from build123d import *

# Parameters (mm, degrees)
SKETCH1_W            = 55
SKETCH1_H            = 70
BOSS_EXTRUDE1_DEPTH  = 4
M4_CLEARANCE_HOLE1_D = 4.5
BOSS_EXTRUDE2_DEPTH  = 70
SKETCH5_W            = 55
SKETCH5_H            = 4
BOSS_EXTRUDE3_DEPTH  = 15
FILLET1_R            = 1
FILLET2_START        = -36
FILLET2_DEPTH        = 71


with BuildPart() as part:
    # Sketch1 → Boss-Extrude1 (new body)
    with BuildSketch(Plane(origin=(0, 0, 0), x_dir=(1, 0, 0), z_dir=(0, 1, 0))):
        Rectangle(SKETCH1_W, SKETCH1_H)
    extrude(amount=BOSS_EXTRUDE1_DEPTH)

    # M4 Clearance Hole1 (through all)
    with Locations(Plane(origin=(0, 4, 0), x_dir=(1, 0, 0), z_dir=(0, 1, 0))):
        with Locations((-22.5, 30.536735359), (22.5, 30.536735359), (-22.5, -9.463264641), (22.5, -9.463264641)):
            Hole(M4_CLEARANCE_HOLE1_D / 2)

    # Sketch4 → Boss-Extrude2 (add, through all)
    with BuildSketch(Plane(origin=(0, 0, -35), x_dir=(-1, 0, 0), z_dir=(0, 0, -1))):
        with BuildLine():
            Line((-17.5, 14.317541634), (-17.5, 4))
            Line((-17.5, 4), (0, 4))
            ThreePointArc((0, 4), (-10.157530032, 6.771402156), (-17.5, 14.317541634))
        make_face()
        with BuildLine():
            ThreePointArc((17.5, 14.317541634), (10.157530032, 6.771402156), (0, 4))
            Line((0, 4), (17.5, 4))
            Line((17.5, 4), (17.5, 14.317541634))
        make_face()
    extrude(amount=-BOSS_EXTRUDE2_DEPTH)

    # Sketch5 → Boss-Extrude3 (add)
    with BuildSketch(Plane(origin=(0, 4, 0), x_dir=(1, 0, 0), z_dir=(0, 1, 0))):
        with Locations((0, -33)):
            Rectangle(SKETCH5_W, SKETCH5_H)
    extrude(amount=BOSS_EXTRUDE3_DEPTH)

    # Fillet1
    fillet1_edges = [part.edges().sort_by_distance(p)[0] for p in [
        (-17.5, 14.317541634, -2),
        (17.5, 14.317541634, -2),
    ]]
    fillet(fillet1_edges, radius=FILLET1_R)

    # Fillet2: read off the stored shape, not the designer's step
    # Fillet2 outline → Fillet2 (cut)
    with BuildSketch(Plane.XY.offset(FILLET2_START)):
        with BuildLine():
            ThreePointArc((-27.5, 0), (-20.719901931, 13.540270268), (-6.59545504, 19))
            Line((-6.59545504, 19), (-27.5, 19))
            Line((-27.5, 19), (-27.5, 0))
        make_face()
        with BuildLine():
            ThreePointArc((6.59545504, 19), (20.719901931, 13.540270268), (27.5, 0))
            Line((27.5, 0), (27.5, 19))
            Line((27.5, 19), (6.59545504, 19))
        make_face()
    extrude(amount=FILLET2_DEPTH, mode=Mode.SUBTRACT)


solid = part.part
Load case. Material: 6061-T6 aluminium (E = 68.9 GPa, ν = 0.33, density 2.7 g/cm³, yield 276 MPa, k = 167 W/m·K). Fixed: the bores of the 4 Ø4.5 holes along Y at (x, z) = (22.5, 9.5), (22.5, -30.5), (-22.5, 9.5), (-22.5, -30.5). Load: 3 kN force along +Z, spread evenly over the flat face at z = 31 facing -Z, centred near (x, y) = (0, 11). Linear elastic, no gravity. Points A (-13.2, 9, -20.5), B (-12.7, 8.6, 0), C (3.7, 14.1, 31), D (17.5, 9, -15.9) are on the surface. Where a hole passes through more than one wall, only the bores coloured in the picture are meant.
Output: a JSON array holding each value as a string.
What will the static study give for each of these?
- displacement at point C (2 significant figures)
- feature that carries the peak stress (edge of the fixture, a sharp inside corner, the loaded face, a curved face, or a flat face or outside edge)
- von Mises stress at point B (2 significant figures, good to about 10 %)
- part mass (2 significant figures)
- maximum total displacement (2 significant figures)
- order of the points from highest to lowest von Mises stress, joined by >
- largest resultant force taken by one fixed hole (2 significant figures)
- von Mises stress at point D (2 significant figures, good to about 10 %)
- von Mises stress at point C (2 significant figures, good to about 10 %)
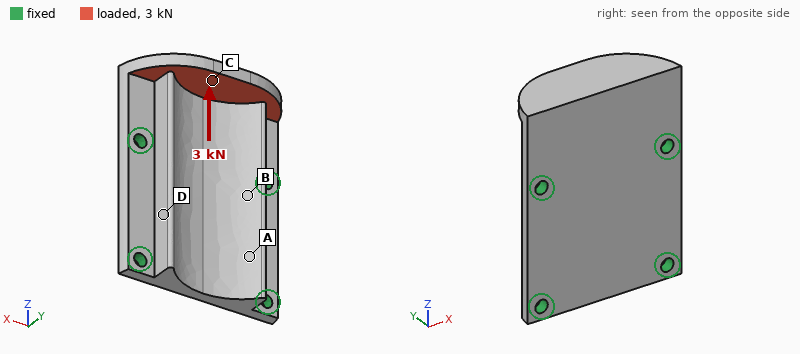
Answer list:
["0.12 mm", "a curved face", "33 MPa", "65 g", "0.19 mm", "C > B > D > A", "830 N", "18 MPa", "47 MPa"]
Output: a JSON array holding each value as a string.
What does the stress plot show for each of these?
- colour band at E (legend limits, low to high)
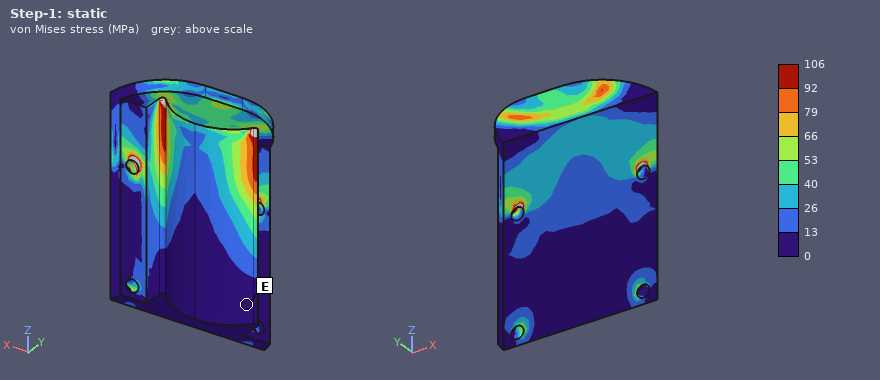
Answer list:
["0 to 13 MPa"]
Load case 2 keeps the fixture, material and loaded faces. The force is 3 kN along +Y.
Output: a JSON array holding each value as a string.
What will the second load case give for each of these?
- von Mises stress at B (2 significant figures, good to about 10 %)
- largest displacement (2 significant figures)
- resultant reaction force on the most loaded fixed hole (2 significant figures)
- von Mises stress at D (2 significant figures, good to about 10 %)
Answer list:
["70 MPa", "0.26 mm", "2.5 kN", "41 MPa"]
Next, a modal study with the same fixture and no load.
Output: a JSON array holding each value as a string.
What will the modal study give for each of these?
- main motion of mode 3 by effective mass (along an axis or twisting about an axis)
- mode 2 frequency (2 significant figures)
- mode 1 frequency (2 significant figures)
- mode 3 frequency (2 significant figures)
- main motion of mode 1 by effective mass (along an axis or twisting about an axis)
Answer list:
["along Y", "7700 Hz", "4600 Hz", "8500 Hz", "along Y"]
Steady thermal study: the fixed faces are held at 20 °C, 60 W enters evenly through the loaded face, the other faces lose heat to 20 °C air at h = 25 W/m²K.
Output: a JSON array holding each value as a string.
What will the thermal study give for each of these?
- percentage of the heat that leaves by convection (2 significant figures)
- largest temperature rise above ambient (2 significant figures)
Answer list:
["5.7 %", "49 K"]
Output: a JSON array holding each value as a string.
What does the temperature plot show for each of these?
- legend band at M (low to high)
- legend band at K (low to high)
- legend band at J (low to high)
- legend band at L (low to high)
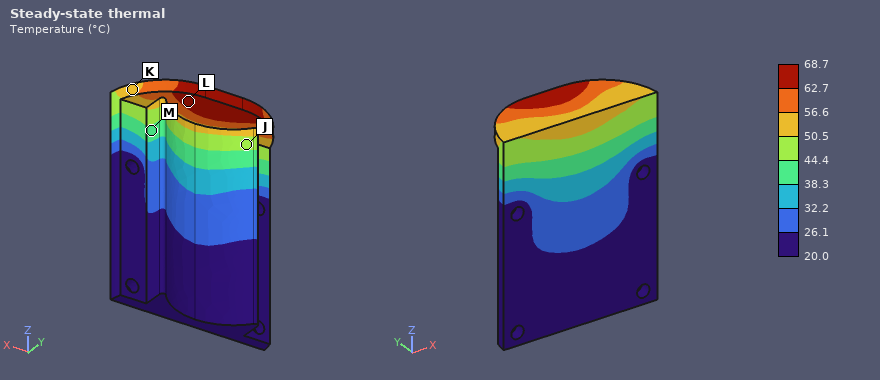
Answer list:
["38.3 to 44.4 °C", "50.5 to 56.6 °C", "44.4 to 50.5 °C", "62.7 to 68.7 °C"]
